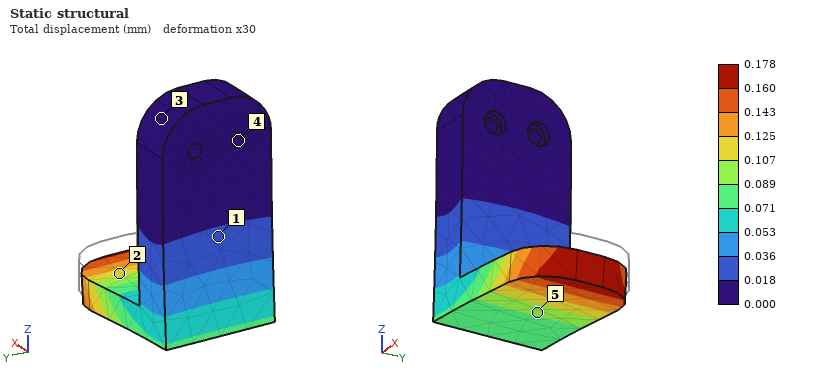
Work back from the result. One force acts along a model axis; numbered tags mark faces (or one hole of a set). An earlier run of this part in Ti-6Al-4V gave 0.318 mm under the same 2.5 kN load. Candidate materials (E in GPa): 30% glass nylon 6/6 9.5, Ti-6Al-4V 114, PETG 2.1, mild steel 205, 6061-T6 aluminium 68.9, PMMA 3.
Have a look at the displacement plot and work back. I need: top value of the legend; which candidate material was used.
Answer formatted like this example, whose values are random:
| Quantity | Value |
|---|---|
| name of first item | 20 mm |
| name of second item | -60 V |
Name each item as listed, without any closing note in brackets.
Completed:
| Quantity | Value |
|---|---|
| top value of the legend | 0.178 mm |
| which candidate material was used | mild steel |
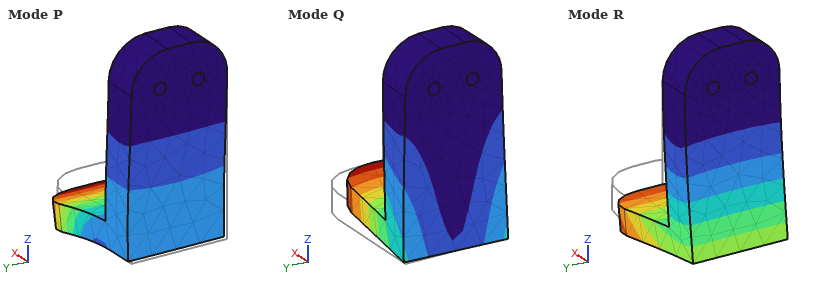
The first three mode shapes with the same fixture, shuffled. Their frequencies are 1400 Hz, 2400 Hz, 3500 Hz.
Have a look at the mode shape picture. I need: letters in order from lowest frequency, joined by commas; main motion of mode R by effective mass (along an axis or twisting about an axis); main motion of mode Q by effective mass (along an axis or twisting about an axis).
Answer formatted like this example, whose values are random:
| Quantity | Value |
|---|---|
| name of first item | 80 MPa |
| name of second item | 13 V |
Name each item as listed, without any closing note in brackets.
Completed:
| Quantity | Value |
|---|---|
| letters in order from lowest frequency, joined by commas | R, Q, P |
| main motion of mode R by effective mass | along X |
| main motion of mode Q by effective mass | along Y |
